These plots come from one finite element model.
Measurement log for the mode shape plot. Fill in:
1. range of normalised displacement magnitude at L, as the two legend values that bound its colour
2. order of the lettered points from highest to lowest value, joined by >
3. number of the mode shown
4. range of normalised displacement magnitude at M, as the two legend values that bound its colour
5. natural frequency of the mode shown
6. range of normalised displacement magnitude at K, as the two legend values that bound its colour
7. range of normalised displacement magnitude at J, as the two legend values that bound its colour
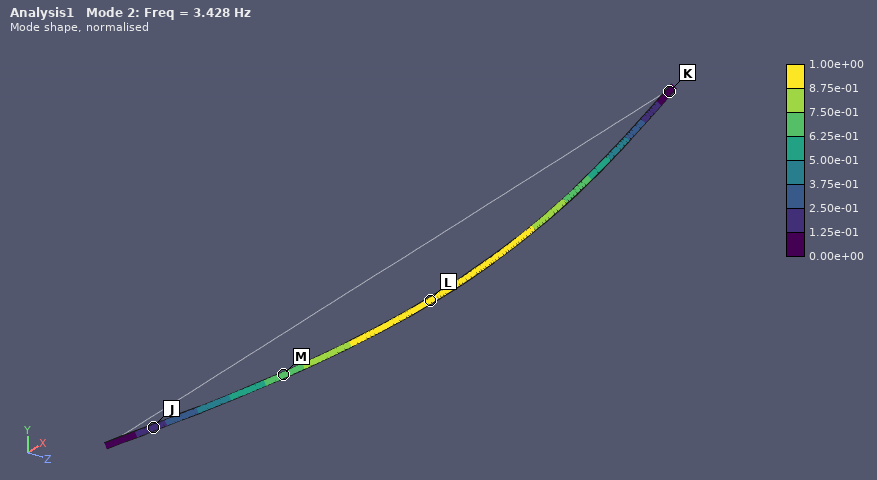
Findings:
8.75e-01 to 1.00e+00
L > M > J > K
2
6.25e-01 to 7.50e-01
3.428 Hz
0.00e+00 to 1.25e-01
1.25e-01 to 2.50e-01
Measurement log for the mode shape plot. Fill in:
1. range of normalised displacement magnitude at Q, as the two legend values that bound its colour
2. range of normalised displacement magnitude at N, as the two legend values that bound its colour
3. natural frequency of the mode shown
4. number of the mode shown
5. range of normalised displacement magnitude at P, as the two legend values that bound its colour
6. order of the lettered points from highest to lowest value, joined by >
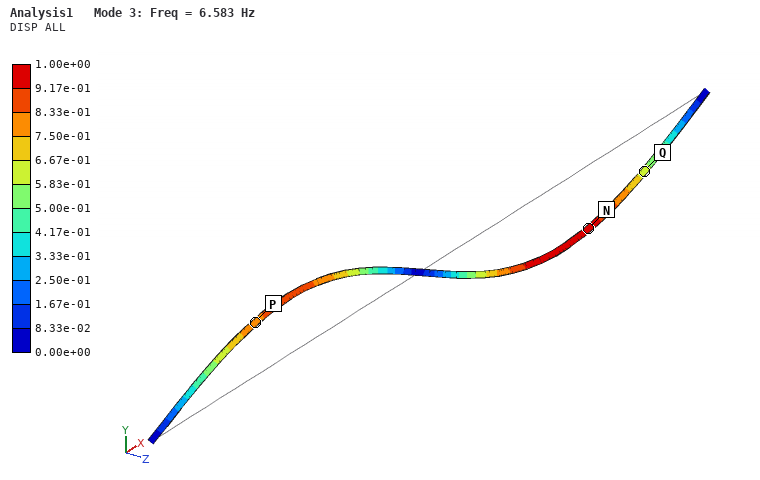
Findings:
5.83e-01 to 6.67e-01
9.17e-01 to 1.00e+00
6.583 Hz
3
7.50e-01 to 8.33e-01
N > P > Q
